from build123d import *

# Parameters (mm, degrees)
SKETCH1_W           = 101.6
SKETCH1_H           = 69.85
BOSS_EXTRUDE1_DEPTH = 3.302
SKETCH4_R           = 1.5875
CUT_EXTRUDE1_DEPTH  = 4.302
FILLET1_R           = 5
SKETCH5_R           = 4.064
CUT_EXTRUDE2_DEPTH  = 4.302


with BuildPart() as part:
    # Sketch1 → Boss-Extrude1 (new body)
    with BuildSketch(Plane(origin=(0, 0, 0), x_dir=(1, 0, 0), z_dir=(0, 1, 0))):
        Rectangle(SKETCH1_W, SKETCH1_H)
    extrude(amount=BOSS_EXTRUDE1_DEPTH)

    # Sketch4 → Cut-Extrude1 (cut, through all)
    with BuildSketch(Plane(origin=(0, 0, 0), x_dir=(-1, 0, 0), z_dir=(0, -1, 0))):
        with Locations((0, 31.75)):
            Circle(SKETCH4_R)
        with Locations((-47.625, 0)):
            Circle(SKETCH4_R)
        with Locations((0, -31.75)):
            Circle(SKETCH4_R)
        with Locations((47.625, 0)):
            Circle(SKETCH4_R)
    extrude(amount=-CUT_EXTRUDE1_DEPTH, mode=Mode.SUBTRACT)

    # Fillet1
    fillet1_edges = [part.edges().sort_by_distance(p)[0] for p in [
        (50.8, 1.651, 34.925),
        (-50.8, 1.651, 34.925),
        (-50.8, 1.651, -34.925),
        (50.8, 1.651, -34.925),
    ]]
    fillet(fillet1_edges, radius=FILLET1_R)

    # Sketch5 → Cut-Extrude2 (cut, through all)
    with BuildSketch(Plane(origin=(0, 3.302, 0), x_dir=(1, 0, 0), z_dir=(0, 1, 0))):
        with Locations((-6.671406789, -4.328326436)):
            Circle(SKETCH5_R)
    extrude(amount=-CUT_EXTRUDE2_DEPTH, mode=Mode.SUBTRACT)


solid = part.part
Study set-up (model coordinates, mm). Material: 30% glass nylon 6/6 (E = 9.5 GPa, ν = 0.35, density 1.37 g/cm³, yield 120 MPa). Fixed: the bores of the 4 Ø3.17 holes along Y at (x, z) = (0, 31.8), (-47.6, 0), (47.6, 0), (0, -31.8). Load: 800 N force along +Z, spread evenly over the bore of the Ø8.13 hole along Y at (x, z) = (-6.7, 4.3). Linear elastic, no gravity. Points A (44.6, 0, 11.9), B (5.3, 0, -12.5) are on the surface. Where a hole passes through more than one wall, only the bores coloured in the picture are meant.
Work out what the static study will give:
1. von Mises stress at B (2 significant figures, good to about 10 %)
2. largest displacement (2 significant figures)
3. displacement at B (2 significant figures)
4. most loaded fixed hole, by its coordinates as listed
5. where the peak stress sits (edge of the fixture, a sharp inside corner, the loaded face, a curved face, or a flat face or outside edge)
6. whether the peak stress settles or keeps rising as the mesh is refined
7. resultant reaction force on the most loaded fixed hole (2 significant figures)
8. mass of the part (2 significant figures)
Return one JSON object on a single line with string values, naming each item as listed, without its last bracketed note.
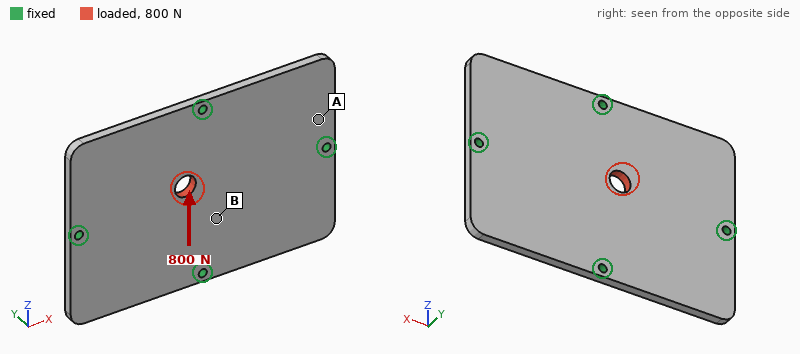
{"von Mises stress at B": "3.1 MPa", "largest displacement": "24 µm", "displacement at B": "10 µm", "most loaded fixed hole, by its coordinates as listed": "(0, 31.8)", "where the peak stress sits": "edge of the fixture", "whether the peak stress settles or keeps rising as the mesh is refined": "keeps rising", "resultant reaction force on the most loaded fixed hole": "330 N", "mass of the part": "32 g"}
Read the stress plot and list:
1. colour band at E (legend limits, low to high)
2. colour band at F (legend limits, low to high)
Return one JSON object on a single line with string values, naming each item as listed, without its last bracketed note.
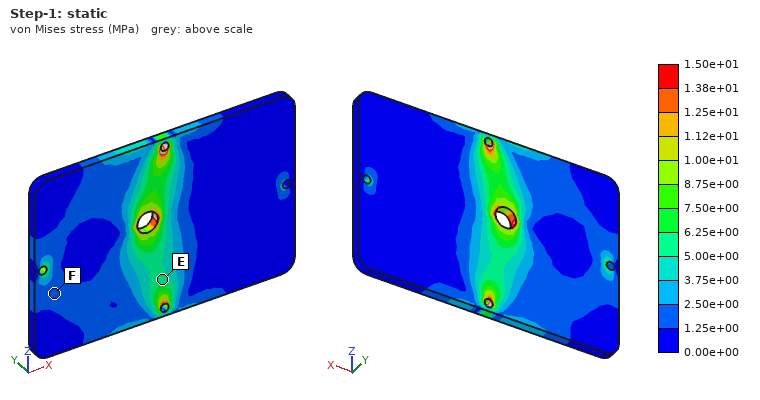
{"colour band at E": "5.00e+00 to 6.25e+00 MPa", "colour band at F": "1.25e+00 to 2.50e+00 MPa"}
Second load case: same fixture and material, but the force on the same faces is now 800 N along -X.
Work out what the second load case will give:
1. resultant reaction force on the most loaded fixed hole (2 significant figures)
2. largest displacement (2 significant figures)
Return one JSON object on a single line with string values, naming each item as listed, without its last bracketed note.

{"resultant reaction force on the most loaded fixed hole": "240 N", "largest displacement": "23 µm"}
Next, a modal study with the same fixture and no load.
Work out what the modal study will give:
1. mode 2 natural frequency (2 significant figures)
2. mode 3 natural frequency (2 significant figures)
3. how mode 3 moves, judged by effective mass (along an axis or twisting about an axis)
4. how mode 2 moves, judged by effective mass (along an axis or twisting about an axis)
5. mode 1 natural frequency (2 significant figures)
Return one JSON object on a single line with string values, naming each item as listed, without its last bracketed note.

{"mode 2 natural frequency": "1500 Hz", "mode 3 natural frequency": "1700 Hz", "how mode 3 moves, judged by effective mass": "twisting about Z", "how mode 2 moves, judged by effective mass": "twisting about X", "mode 1 natural frequency": "1500 Hz"}
